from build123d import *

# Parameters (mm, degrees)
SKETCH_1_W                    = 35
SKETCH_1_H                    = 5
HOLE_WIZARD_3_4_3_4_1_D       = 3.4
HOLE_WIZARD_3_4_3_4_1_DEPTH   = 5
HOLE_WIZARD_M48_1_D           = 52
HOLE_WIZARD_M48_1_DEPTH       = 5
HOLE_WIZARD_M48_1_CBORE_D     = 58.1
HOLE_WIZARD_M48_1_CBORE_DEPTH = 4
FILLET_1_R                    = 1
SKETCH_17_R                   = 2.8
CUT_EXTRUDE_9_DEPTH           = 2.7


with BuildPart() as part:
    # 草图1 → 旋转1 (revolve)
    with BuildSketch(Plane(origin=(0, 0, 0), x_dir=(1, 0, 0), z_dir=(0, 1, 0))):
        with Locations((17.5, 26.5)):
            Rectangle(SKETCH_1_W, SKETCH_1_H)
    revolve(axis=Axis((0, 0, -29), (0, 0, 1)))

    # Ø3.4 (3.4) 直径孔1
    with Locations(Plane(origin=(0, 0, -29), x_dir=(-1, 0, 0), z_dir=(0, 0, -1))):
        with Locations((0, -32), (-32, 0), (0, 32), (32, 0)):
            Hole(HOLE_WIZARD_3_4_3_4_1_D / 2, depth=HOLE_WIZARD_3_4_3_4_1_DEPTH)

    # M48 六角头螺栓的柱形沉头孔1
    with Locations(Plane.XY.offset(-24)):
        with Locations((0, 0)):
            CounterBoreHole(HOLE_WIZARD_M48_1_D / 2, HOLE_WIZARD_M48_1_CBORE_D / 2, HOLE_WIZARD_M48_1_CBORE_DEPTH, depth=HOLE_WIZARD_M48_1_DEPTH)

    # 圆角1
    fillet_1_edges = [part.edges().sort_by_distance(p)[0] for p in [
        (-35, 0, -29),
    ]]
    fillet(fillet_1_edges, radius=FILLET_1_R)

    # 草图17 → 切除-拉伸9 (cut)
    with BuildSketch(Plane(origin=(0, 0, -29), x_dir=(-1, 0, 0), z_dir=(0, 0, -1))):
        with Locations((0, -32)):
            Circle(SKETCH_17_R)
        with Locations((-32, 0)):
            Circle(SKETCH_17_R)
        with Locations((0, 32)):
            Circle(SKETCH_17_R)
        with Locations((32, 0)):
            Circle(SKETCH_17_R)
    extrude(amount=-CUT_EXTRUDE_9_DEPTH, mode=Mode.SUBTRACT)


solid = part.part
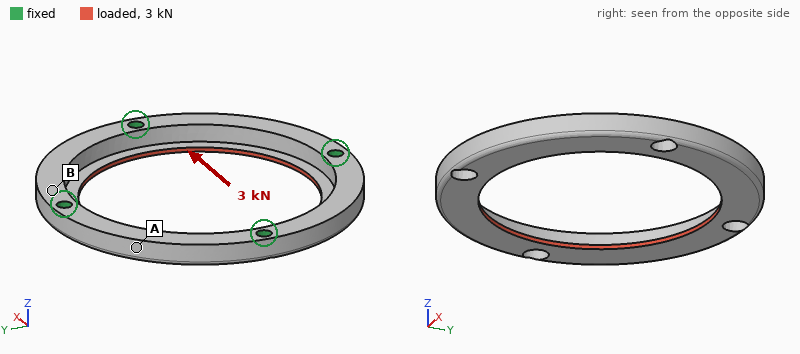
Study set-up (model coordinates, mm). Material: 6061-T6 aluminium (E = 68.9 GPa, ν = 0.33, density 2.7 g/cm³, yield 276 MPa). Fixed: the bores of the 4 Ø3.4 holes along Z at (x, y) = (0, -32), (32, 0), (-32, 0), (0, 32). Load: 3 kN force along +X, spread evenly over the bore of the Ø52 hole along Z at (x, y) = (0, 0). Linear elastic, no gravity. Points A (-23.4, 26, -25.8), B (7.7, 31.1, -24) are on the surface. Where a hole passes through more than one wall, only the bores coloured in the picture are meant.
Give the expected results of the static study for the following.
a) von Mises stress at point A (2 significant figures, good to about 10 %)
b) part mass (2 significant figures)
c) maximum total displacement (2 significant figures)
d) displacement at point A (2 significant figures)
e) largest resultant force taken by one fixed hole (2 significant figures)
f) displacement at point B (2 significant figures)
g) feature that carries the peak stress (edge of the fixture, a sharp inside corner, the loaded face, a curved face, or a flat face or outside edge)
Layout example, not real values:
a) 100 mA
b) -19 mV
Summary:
a) 15 MPa
b) 17 g
c) 34 µm
d) 31 µm
e) 1.0 kN
f) 10 µm
g) a curved face
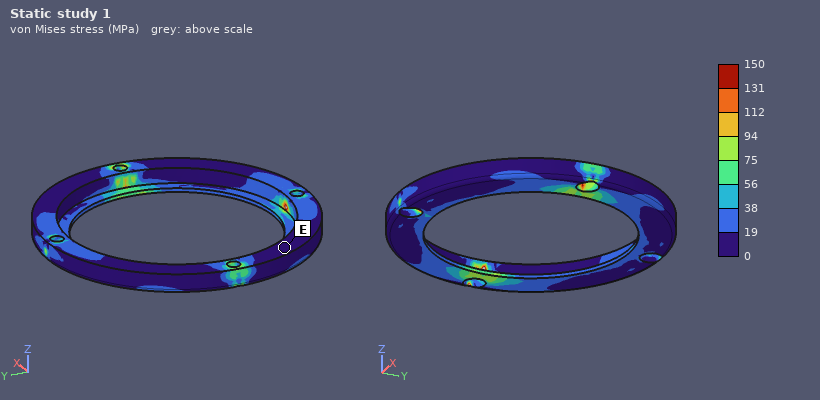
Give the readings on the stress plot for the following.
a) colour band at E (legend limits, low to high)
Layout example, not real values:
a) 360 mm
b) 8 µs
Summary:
a) 0 to 19 MPa
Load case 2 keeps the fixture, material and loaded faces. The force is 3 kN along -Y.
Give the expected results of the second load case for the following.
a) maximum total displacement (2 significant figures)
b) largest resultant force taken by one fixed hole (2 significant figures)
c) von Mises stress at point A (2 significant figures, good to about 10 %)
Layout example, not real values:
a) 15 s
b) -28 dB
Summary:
a) 34 µm
b) 1.0 kN
c) 16 MPa
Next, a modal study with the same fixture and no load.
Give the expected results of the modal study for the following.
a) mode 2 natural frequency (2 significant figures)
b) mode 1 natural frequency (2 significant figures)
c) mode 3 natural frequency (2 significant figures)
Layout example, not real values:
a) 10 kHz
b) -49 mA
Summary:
a) 7500 Hz
b) 6400 Hz
c) 7500 Hz
